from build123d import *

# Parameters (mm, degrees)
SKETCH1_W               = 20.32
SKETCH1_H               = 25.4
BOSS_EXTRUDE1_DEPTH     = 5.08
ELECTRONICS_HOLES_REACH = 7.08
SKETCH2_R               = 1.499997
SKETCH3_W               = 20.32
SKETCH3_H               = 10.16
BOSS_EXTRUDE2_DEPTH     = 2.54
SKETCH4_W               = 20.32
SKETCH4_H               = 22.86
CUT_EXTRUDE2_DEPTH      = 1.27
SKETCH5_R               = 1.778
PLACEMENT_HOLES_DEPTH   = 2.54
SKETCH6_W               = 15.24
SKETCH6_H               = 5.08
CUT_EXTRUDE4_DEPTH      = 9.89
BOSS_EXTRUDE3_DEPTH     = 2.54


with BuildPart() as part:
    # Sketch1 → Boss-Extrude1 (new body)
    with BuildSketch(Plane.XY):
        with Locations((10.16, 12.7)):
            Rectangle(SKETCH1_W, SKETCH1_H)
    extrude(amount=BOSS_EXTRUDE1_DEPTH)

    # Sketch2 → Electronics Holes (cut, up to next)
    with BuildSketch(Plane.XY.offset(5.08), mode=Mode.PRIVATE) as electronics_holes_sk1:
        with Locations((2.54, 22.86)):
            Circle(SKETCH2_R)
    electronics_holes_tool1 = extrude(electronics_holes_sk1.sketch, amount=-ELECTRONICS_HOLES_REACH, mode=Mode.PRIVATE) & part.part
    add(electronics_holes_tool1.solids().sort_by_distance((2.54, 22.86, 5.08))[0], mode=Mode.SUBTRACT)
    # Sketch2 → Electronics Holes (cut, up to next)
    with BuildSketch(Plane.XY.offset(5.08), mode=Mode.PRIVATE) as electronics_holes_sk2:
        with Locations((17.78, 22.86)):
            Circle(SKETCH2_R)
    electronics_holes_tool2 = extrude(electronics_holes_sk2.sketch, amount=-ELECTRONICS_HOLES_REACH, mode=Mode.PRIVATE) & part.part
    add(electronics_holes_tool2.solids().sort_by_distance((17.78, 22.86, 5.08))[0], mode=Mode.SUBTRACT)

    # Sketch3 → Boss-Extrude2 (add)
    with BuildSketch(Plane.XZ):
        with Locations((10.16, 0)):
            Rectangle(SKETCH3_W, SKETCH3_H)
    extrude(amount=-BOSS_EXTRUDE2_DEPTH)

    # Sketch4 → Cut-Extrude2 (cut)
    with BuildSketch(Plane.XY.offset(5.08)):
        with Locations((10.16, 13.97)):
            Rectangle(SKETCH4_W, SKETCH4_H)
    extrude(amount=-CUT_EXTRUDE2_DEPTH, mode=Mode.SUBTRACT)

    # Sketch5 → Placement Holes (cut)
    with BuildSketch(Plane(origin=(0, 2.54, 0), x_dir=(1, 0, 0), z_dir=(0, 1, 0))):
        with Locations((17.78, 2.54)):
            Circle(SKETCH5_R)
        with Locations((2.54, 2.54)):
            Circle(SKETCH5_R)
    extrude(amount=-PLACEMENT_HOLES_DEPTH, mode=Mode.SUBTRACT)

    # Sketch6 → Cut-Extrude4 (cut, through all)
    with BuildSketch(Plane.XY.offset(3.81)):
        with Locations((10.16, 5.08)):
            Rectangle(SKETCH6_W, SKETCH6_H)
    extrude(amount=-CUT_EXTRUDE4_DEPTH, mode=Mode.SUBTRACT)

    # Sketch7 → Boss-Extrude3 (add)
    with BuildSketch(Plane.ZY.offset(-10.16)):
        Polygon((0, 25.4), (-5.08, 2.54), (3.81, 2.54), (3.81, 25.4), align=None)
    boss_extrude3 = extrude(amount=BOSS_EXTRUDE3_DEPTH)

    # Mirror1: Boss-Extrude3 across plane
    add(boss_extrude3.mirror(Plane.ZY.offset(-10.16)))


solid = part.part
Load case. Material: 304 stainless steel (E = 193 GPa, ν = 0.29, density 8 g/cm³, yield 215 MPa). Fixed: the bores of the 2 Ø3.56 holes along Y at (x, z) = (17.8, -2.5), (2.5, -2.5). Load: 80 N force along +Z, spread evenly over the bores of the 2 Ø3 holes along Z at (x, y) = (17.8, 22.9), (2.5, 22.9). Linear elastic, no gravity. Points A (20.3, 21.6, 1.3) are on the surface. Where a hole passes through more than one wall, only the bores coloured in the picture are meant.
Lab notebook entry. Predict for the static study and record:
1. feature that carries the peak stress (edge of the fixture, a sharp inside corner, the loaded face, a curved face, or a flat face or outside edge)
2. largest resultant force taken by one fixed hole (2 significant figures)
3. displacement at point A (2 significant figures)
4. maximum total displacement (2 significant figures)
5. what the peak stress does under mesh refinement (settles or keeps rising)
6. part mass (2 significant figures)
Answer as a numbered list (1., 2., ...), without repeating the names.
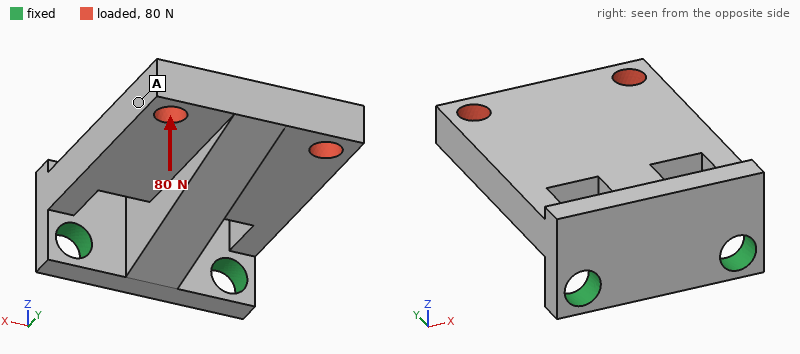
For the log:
1. edge of the fixture
2. 53 N
3. 19 µm
4. 23 µm
5. keeps rising
6. 18 g
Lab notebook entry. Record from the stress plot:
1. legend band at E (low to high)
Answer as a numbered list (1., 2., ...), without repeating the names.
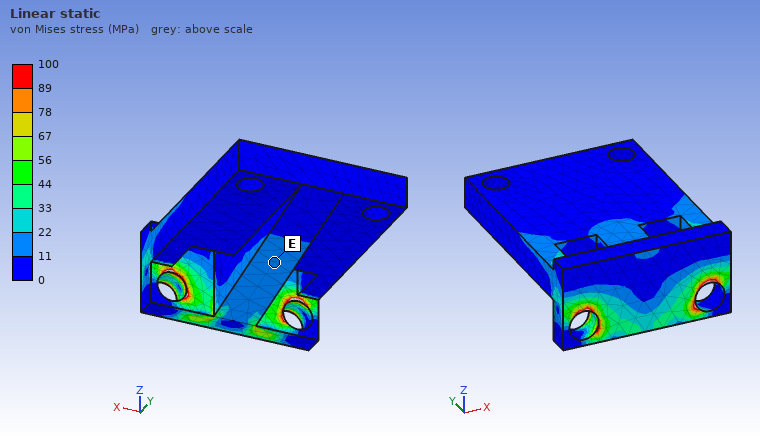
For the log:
1. 11 to 22 MPa
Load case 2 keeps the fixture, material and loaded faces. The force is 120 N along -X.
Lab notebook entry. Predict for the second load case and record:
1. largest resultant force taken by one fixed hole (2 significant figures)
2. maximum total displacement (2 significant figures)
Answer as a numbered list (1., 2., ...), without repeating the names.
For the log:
1. 180 N
2. 4.9 µm
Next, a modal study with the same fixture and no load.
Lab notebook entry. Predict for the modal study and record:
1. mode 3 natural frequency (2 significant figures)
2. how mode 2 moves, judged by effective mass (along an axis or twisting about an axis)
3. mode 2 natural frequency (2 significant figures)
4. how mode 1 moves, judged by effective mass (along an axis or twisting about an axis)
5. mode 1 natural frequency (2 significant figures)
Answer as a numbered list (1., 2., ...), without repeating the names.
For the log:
1. 14 kHz
2. along X
3. 10 kHz
4. along Z
5. 4100 Hz
